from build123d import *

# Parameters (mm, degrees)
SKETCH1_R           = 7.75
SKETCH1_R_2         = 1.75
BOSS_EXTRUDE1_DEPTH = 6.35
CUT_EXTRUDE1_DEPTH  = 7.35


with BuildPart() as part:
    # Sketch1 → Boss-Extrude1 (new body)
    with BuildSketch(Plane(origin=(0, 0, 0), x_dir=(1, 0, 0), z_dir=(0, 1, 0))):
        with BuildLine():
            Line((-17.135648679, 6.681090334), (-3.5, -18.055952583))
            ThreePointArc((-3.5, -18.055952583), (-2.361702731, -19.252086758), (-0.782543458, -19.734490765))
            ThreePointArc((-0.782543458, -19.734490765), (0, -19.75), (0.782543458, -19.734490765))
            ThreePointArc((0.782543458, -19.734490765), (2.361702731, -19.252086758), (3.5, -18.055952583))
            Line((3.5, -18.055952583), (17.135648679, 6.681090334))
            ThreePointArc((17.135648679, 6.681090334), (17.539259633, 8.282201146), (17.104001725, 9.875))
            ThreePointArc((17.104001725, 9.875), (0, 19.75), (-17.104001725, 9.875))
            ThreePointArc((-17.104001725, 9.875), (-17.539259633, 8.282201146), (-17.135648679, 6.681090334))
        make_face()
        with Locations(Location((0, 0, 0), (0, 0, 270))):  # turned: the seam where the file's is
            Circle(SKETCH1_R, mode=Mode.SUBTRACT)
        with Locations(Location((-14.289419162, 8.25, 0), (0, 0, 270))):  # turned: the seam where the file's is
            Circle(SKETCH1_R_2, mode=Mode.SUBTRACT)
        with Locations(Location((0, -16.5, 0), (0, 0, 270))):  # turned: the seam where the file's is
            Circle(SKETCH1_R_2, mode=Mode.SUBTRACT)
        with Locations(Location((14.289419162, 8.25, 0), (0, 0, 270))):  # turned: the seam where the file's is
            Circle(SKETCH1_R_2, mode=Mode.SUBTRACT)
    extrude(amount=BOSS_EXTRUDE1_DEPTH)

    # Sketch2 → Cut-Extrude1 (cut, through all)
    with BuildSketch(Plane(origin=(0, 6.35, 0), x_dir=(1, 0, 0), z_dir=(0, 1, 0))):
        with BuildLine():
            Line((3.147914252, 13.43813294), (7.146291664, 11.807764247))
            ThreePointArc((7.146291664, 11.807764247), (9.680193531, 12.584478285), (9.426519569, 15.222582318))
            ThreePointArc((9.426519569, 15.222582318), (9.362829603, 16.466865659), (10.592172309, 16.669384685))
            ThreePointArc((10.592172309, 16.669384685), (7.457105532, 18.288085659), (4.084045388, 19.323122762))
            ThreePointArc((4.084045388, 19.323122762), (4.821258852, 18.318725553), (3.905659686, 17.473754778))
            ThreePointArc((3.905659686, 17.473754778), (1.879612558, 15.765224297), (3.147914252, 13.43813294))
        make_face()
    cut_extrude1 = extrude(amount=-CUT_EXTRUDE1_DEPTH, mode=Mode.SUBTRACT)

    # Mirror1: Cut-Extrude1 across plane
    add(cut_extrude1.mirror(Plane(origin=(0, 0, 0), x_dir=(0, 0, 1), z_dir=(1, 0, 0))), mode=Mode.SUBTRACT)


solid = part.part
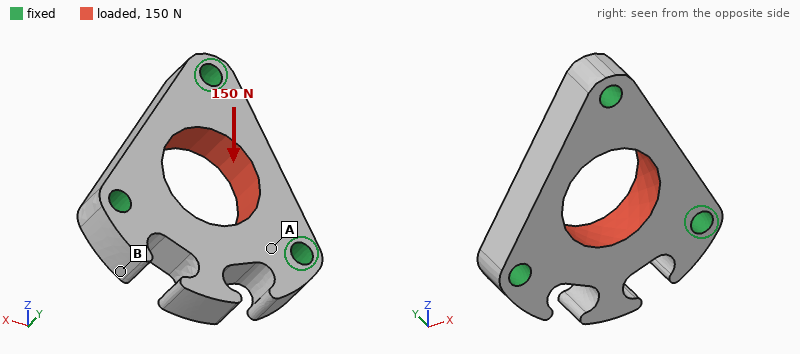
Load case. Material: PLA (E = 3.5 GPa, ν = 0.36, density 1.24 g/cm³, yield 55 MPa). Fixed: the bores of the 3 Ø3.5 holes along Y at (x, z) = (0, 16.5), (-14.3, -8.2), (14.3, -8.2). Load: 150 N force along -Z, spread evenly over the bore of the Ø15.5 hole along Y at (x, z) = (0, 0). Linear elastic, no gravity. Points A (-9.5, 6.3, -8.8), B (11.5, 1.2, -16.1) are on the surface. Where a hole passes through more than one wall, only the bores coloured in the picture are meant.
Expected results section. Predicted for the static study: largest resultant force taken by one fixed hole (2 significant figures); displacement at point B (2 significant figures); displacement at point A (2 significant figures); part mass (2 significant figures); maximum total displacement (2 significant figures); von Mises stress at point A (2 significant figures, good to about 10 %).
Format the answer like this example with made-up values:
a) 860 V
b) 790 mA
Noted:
a) 51 N
b) 5.4 µm
c) 4.0 µm
d) 4.5 g
e) 11 µm
f) 1.3 MPa
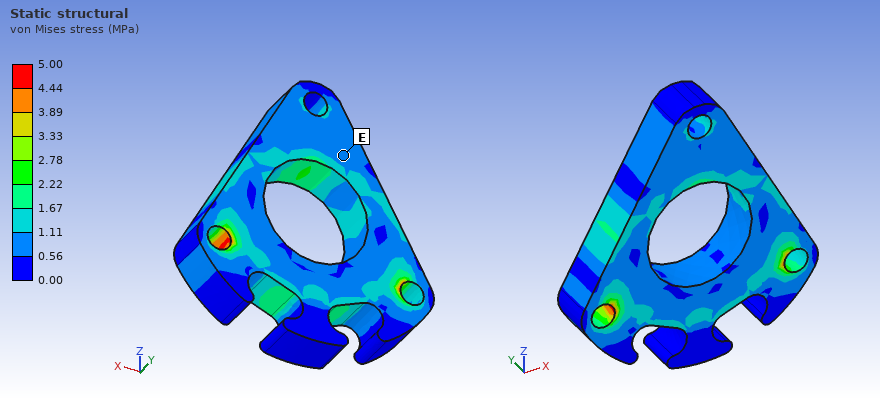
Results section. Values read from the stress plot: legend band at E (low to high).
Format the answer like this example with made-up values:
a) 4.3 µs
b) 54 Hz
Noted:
a) 0.56 to 1.11 MPa
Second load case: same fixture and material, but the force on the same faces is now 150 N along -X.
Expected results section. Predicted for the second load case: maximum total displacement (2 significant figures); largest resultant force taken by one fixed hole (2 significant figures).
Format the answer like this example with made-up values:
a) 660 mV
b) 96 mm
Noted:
a) 13 µm
b) 52 N
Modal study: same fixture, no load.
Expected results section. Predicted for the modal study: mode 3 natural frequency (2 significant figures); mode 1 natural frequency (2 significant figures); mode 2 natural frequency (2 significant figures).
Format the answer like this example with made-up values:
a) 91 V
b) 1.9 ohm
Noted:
a) 11 kHz
b) 6400 Hz
c) 10 kHz
